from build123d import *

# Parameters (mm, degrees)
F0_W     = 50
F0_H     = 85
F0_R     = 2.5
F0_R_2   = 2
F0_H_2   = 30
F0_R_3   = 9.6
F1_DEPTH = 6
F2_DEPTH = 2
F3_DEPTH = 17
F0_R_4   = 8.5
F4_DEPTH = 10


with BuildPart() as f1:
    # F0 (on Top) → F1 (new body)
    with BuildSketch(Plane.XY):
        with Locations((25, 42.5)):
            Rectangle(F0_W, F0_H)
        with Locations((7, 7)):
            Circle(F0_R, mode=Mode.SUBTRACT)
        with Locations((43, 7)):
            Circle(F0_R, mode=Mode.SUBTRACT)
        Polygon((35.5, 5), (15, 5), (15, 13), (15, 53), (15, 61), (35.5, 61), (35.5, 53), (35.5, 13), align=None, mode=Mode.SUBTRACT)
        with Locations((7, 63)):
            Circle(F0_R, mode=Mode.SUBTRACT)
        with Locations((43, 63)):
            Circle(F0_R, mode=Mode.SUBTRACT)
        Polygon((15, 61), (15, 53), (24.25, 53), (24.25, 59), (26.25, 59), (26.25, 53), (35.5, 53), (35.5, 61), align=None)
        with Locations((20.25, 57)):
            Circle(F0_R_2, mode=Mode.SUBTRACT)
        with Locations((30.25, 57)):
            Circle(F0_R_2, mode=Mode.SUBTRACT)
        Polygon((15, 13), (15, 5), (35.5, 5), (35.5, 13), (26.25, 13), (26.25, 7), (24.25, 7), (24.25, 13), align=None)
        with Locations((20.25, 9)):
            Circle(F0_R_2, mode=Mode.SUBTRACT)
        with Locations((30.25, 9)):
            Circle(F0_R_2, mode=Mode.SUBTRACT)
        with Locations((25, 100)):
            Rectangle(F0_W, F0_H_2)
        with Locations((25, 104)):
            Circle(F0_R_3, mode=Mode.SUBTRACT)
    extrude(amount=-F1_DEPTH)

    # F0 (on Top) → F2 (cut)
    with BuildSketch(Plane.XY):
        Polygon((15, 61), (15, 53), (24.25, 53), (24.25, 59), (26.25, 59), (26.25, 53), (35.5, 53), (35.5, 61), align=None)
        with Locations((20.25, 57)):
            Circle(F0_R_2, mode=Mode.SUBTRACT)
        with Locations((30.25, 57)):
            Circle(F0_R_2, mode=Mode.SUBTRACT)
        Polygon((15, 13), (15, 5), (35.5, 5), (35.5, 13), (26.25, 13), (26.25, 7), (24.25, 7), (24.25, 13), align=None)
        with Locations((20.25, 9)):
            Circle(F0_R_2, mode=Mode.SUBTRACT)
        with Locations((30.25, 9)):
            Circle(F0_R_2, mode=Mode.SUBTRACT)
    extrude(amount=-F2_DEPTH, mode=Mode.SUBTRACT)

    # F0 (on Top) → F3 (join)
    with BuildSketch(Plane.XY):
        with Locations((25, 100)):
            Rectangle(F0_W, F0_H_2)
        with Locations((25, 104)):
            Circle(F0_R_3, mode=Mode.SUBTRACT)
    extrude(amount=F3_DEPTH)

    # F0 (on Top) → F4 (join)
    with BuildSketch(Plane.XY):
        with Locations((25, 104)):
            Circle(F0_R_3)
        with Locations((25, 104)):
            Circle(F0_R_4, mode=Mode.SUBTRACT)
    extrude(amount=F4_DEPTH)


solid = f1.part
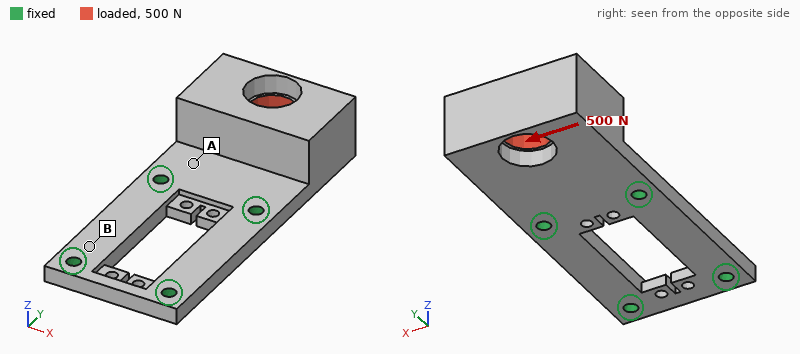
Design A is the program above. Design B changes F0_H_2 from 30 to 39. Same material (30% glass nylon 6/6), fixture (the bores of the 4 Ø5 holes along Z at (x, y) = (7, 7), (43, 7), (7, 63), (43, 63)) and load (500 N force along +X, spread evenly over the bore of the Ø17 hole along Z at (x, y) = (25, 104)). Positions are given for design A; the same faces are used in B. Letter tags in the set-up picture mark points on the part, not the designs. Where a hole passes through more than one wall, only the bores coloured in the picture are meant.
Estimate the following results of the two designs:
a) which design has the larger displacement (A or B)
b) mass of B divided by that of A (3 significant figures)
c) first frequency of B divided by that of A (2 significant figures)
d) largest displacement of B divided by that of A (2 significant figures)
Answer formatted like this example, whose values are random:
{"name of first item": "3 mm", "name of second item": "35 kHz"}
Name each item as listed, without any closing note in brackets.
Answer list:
{"which design has the larger displacement": "A", "mass of B divided by that of A": "1.19", "first frequency of B divided by that of A": "0.86", "largest displacement of B divided by that of A": "0.76"}
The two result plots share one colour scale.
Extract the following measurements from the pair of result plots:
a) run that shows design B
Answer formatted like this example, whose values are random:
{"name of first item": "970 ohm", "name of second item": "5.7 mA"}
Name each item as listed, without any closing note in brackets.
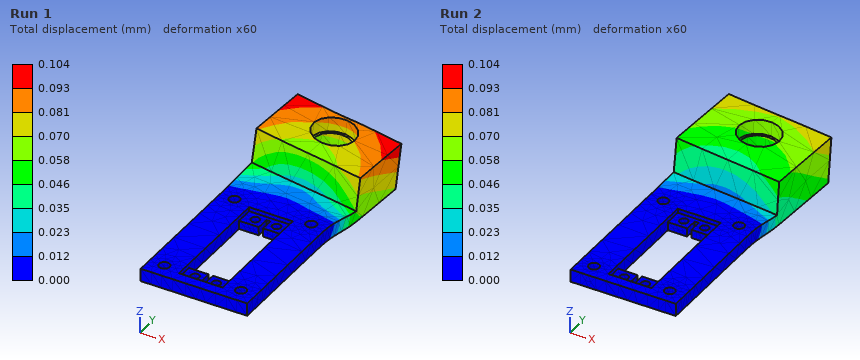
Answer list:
{"run that shows design B": "Run 2"}
